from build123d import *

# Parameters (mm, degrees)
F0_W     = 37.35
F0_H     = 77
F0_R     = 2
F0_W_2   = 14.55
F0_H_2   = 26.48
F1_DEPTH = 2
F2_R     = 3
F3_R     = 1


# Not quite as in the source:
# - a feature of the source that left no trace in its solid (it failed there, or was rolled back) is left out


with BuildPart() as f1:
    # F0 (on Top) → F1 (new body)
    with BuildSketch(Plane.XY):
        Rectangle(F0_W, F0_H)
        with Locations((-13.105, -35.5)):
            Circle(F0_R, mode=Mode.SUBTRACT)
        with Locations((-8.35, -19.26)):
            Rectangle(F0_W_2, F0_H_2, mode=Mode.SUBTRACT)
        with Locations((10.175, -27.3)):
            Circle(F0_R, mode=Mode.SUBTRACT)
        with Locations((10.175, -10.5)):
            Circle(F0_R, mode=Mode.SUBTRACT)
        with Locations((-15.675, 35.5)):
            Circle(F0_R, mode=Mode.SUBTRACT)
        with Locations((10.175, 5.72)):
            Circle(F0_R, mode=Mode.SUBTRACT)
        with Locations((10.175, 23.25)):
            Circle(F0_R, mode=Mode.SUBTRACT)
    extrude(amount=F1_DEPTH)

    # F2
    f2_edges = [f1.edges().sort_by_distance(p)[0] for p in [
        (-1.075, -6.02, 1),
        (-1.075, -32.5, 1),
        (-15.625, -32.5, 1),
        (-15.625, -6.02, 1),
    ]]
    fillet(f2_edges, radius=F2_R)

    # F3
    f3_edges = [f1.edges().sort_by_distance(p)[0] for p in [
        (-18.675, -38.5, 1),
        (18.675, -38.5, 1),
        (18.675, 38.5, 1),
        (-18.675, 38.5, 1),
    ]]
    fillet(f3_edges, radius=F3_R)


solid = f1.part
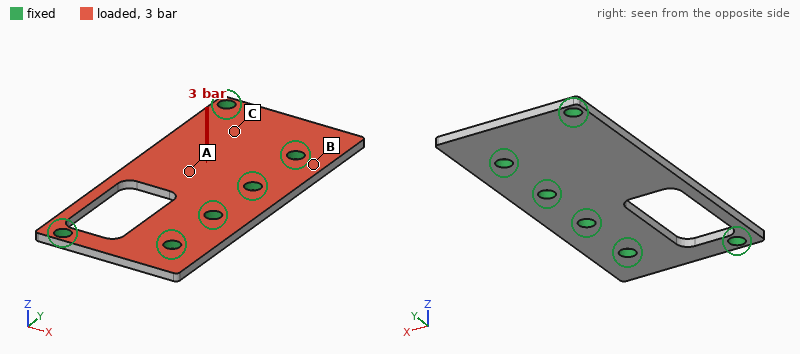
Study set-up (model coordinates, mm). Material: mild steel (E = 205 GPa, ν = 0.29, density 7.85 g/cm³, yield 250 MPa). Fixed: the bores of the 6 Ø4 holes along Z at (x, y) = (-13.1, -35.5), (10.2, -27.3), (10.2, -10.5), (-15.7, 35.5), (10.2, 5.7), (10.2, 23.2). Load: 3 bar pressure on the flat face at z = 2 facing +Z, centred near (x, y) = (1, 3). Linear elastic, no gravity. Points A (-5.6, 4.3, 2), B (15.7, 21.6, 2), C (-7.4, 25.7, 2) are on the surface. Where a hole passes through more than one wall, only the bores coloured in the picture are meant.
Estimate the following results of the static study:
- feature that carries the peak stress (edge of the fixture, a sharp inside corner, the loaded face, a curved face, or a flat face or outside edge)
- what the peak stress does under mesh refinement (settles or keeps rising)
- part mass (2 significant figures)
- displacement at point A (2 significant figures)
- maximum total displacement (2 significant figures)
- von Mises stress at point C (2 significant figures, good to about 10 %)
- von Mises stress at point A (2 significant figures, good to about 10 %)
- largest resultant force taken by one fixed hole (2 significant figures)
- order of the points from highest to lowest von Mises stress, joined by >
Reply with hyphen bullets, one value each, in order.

- edge of the fixture
- keeps rising
- 38 g
- 29 µm
- 72 µm
- 40 MPa
- 21 MPa
- 160 N
- C > A > B
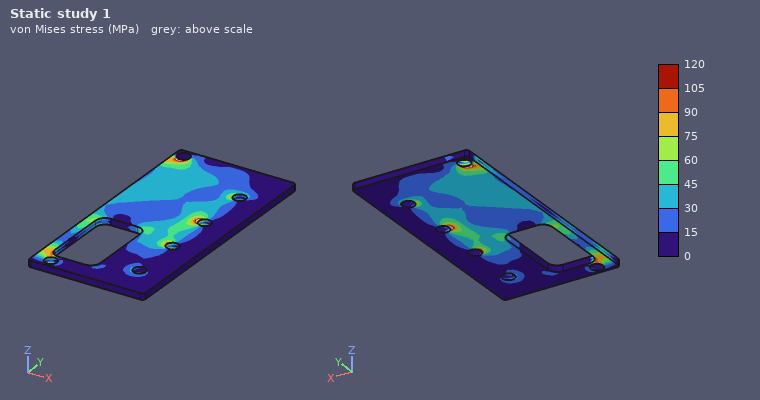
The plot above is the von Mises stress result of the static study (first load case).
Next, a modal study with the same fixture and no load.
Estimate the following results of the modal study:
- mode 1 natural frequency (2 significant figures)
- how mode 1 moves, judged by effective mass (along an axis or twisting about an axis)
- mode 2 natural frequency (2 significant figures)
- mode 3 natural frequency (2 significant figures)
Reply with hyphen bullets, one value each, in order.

- 3400 Hz
- along Z
- 7400 Hz
- 8800 Hz
